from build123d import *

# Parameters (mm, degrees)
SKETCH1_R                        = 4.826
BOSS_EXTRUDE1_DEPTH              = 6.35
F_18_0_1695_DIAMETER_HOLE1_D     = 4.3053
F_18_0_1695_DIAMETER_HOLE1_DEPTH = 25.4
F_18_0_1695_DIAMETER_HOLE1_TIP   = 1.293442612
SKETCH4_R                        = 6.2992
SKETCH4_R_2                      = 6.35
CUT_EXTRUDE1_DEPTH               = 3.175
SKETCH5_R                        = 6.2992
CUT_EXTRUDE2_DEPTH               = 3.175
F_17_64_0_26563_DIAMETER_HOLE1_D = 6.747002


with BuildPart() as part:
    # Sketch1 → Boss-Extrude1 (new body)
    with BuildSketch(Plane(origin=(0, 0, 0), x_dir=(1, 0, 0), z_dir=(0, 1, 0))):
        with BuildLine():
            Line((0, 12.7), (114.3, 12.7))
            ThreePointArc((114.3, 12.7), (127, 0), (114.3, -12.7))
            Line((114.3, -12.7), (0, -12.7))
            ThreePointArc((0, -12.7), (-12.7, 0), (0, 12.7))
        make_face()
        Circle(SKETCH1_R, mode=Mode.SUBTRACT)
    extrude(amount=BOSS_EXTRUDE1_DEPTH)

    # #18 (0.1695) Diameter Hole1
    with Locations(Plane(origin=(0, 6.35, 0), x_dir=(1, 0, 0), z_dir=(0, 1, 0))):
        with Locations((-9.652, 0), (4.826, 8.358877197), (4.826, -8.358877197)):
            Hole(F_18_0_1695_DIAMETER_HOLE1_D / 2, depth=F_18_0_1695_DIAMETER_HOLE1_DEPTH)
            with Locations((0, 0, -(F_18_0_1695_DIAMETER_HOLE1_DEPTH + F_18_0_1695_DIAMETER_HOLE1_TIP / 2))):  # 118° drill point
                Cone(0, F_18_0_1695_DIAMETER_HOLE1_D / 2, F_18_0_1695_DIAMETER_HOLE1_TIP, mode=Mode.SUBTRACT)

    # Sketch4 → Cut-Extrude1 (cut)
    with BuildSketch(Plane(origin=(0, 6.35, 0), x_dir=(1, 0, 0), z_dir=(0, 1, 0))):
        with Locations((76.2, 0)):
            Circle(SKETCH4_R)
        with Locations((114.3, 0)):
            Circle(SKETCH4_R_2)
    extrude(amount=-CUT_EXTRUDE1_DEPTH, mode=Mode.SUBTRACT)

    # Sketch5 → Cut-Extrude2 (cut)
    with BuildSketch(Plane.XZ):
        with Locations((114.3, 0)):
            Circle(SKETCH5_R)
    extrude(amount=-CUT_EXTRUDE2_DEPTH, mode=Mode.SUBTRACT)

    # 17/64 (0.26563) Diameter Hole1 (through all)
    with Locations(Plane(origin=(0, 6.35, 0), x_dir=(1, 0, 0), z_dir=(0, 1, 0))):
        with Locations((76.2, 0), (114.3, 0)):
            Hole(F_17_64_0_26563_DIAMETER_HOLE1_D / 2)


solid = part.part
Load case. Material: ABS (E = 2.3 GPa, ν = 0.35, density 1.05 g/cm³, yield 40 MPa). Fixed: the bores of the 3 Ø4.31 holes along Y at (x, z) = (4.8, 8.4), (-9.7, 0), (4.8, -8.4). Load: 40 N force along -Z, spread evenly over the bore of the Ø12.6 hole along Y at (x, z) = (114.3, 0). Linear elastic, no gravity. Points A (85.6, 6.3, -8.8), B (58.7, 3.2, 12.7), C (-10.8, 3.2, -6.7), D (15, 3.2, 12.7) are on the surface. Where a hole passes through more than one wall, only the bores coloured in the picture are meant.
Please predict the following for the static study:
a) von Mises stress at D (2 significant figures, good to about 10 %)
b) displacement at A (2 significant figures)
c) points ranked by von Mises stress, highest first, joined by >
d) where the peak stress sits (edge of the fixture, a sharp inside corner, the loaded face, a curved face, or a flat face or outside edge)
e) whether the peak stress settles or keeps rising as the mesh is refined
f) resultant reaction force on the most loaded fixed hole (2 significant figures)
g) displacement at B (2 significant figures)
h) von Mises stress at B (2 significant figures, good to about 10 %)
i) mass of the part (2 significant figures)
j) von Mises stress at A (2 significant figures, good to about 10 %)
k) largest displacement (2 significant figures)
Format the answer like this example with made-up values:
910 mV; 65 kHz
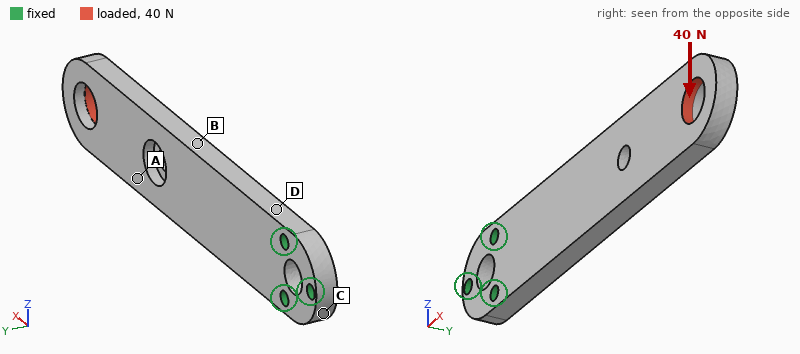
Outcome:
5.7 MPa; 0.56 mm; D > B > A > C; edge of the fixture; keeps rising; 240 N; 0.30 mm; 3.3 MPa; 21 g; 1.2 MPa; 1.1 mm
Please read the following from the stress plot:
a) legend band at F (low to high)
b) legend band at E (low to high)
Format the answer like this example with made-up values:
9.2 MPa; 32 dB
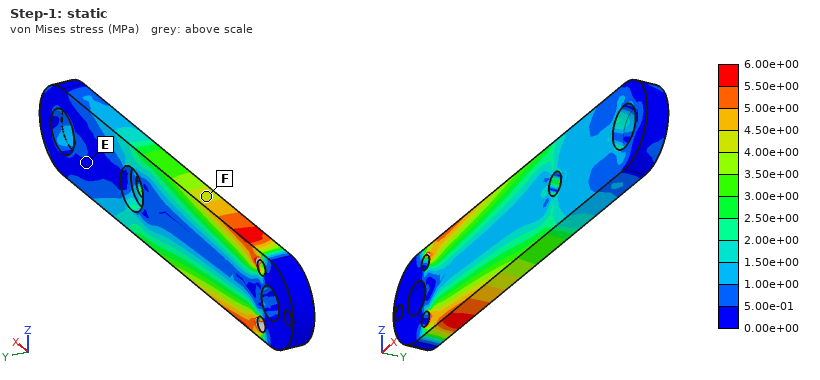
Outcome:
4.00e+00 to 4.50e+00 MPa; 0.00e+00 to 5.00e-01 MPa
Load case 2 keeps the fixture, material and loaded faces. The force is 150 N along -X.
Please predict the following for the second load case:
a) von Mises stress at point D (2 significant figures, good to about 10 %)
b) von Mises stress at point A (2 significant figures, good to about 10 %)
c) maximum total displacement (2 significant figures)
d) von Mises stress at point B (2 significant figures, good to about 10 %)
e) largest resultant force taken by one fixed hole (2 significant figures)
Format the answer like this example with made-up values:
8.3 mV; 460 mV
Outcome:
0.96 MPa; 0.38 MPa; 1.5 mm; 1.0 MPa; 76 N
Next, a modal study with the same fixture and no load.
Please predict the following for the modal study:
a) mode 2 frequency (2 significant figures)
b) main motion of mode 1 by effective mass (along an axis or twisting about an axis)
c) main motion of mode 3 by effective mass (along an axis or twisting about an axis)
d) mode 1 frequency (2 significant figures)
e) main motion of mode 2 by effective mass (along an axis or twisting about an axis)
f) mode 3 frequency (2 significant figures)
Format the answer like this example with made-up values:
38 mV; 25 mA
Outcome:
450 Hz; along Y; along Y; 110 Hz; along Z; 650 Hz
